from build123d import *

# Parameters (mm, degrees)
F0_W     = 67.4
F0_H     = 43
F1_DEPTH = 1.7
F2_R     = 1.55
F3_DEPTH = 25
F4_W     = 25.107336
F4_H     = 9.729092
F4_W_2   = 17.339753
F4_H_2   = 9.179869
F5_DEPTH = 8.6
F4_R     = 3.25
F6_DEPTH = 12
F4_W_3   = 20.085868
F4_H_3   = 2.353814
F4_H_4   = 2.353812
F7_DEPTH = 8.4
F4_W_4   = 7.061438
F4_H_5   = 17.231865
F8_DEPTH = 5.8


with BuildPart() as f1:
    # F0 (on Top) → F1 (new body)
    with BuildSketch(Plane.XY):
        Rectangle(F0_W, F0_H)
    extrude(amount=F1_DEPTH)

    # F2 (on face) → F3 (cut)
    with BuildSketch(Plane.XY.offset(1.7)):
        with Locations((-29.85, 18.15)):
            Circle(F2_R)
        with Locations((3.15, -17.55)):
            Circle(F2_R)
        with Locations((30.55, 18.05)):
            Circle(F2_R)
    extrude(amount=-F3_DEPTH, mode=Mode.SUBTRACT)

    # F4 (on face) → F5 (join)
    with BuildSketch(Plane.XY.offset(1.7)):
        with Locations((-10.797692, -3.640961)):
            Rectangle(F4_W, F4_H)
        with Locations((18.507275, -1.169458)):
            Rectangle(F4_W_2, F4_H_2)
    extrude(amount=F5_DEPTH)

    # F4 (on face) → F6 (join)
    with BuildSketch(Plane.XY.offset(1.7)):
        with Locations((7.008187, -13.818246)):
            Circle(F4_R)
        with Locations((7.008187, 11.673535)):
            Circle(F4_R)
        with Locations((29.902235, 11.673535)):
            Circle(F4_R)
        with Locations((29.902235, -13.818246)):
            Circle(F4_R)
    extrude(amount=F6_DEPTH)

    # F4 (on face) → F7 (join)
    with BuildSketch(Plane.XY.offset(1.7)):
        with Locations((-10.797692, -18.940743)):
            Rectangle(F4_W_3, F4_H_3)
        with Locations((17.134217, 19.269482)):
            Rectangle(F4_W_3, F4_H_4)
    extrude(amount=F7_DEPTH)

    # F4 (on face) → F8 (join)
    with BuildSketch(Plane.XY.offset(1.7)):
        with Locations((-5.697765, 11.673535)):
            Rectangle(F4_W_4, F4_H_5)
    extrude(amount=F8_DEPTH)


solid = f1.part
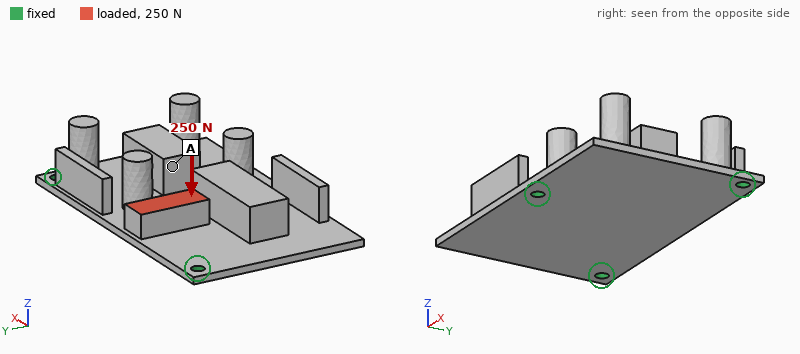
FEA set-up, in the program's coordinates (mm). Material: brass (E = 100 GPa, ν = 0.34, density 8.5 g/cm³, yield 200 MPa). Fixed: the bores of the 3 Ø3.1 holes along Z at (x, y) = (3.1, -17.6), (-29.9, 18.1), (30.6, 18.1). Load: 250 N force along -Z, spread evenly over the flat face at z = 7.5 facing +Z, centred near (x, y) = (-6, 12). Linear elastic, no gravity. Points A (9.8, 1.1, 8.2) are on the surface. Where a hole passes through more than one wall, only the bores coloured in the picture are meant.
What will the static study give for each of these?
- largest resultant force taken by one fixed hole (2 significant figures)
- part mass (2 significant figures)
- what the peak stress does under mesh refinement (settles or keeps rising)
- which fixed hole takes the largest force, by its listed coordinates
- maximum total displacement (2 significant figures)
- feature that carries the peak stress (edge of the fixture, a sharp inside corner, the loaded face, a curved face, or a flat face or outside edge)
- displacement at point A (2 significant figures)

130 N
97 g
keeps rising
(-29.9, 18.1)
0.16 mm
edge of the fixture
0.055 mm
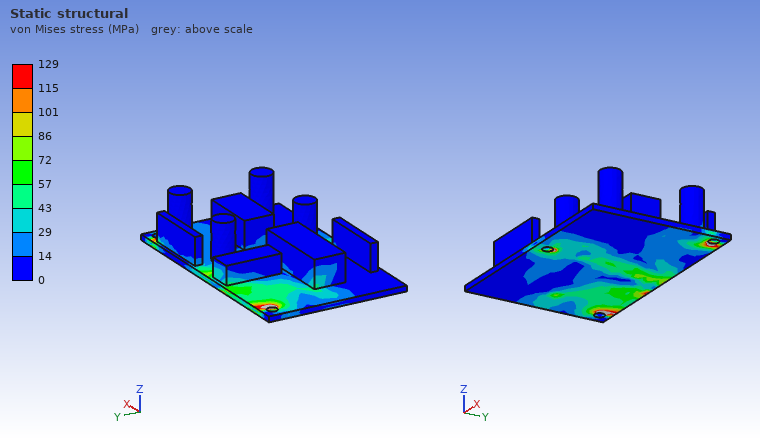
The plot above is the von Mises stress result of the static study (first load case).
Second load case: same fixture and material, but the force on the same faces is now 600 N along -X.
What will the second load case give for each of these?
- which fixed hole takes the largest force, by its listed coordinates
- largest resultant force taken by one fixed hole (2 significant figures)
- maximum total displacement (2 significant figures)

(-29.9, 18.1)
250 N
0.13 mm
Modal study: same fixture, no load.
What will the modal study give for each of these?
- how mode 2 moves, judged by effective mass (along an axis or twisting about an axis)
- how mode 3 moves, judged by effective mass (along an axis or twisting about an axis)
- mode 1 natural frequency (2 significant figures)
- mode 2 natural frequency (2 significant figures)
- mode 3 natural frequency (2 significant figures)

twisting about Y
along Z
1300 Hz
1400 Hz
1700 Hz
